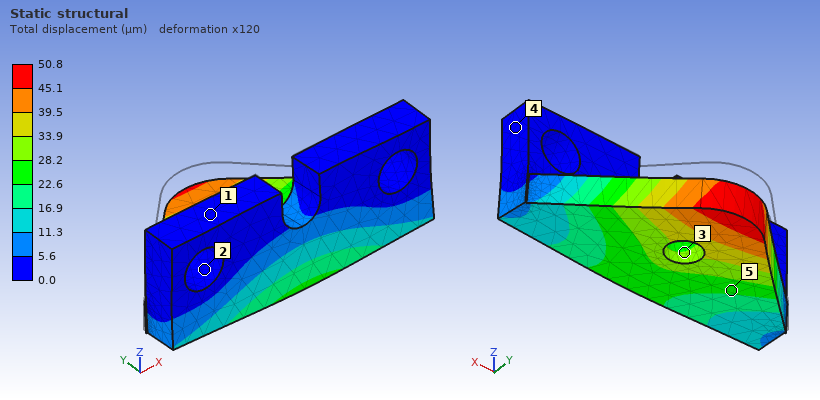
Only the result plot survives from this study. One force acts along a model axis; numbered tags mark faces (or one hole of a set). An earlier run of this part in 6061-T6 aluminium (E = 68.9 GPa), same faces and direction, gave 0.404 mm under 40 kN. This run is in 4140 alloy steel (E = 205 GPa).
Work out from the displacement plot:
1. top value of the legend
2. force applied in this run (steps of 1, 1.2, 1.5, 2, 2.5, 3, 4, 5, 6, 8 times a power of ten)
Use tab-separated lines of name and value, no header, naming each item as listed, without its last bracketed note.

top value of the legend	50.8 µm
force applied in this run	15 kN
